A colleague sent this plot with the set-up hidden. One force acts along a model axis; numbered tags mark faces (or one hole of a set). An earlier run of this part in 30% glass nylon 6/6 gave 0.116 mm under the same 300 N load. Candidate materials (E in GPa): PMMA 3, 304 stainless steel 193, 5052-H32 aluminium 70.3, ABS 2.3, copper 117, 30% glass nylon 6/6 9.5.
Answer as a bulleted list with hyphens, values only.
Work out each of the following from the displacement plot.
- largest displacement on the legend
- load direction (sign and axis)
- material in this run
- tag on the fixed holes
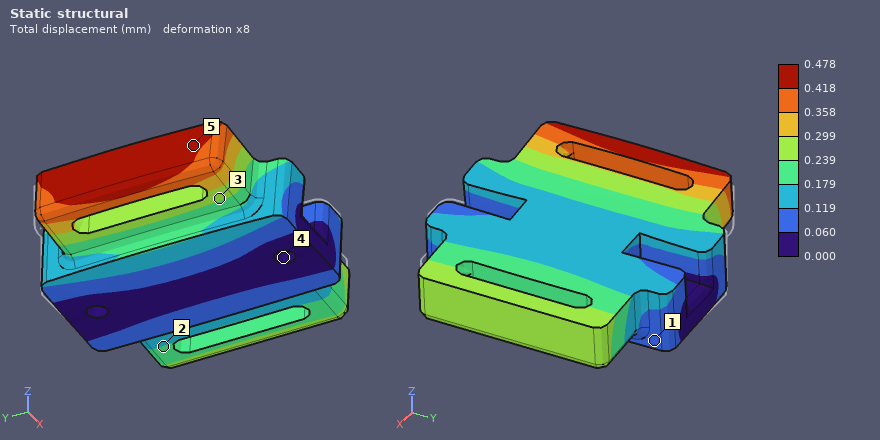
- 0.478 mm
- +Z
- ABS
- 4
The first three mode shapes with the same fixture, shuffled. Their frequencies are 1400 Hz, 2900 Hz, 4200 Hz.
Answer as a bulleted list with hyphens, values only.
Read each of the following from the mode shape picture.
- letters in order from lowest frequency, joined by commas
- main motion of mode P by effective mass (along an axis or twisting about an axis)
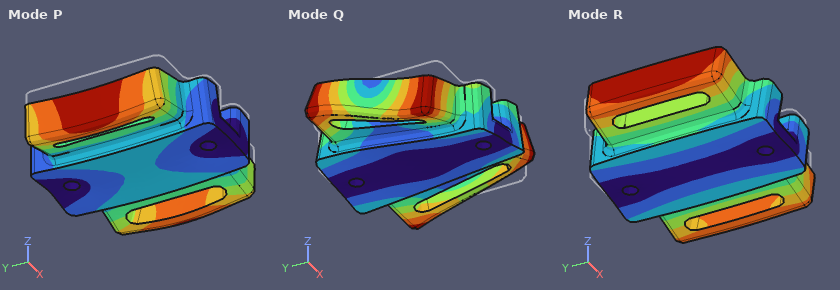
- R, P, Q
- along Z
